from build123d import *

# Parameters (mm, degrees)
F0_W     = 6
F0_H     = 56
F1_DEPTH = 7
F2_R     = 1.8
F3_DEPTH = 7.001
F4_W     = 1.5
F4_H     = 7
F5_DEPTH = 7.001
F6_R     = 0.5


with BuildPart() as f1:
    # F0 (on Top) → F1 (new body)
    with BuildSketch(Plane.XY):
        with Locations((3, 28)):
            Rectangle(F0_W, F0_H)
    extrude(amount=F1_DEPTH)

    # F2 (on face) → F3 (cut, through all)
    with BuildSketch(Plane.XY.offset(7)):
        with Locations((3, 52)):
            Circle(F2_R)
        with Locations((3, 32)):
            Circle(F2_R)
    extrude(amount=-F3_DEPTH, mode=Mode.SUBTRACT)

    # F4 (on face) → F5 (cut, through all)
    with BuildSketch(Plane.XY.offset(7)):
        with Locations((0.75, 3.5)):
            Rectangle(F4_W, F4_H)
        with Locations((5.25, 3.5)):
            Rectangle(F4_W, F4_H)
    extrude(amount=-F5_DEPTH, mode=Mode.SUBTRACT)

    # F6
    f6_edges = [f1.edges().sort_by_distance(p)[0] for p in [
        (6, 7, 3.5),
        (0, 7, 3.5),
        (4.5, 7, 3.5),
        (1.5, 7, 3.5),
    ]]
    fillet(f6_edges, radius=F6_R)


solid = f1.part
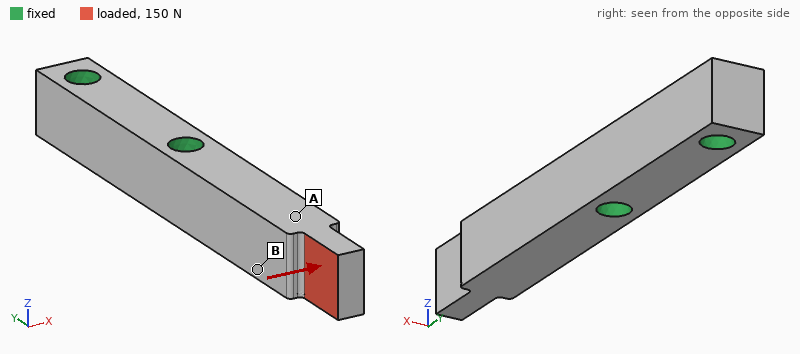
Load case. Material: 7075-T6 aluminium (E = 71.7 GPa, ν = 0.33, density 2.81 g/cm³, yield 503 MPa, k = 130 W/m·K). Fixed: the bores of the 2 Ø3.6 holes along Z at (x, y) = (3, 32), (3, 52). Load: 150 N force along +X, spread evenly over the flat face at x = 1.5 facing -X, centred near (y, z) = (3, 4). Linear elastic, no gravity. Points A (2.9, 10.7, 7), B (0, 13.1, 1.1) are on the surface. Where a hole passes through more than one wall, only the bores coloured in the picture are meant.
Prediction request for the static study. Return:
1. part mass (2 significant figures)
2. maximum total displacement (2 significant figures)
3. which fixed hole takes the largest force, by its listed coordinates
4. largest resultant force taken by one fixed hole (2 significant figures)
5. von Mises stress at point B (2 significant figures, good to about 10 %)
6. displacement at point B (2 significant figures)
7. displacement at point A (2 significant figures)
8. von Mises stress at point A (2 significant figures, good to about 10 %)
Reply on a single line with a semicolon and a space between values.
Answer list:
5.8 g; 0.16 mm; (3, 32); 170 N; 35 MPa; 0.069 mm; 0.081 mm; 9.5 MPa
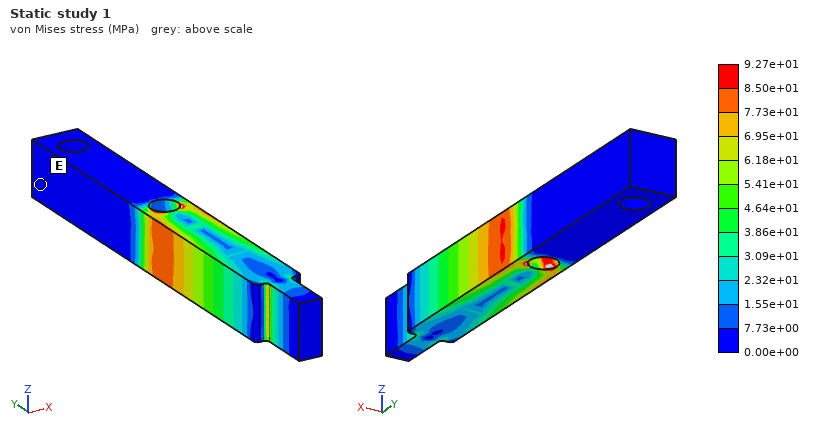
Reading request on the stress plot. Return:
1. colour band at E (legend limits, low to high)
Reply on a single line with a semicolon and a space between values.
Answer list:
0.00e+00 to 7.73e+00 MPa
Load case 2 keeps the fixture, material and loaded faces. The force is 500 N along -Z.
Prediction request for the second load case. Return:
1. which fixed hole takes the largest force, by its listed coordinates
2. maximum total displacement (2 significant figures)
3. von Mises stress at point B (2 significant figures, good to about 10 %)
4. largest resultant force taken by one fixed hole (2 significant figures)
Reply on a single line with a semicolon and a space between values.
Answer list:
(3, 32); 0.37 mm; 77 MPa; 510 N
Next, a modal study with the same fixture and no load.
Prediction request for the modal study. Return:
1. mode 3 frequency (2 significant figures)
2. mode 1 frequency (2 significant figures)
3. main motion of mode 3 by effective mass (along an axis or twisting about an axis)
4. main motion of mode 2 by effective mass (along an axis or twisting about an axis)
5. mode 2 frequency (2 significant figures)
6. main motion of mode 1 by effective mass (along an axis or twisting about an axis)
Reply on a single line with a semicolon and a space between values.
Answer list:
27 kHz; 5700 Hz; twisting about Y; along Z; 7000 Hz; along X
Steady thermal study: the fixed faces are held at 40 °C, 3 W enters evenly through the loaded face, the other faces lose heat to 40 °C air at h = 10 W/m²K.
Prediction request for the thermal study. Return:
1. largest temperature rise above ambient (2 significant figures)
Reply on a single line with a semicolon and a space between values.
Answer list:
18 K
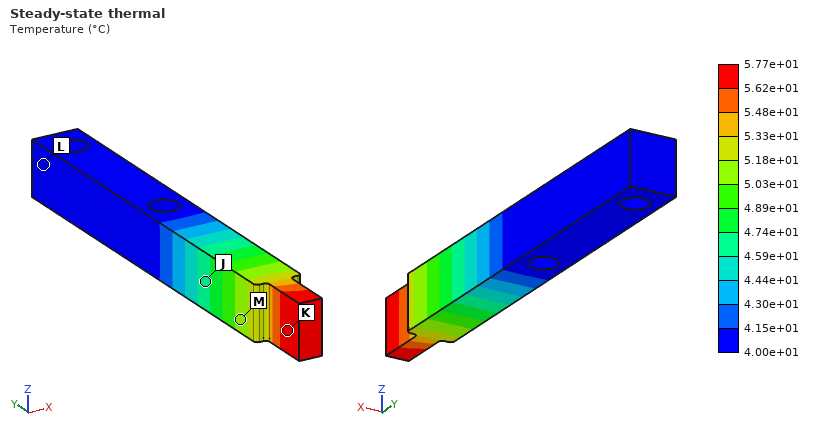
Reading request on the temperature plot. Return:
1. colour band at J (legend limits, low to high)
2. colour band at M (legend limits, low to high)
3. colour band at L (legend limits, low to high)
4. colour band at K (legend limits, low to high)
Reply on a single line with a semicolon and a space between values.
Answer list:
4.59e+01 to 4.74e+01 °C; 5.03e+01 to 5.18e+01 °C; 4.00e+01 to 4.15e+01 °C; 5.62e+01 to 5.77e+01 °C
